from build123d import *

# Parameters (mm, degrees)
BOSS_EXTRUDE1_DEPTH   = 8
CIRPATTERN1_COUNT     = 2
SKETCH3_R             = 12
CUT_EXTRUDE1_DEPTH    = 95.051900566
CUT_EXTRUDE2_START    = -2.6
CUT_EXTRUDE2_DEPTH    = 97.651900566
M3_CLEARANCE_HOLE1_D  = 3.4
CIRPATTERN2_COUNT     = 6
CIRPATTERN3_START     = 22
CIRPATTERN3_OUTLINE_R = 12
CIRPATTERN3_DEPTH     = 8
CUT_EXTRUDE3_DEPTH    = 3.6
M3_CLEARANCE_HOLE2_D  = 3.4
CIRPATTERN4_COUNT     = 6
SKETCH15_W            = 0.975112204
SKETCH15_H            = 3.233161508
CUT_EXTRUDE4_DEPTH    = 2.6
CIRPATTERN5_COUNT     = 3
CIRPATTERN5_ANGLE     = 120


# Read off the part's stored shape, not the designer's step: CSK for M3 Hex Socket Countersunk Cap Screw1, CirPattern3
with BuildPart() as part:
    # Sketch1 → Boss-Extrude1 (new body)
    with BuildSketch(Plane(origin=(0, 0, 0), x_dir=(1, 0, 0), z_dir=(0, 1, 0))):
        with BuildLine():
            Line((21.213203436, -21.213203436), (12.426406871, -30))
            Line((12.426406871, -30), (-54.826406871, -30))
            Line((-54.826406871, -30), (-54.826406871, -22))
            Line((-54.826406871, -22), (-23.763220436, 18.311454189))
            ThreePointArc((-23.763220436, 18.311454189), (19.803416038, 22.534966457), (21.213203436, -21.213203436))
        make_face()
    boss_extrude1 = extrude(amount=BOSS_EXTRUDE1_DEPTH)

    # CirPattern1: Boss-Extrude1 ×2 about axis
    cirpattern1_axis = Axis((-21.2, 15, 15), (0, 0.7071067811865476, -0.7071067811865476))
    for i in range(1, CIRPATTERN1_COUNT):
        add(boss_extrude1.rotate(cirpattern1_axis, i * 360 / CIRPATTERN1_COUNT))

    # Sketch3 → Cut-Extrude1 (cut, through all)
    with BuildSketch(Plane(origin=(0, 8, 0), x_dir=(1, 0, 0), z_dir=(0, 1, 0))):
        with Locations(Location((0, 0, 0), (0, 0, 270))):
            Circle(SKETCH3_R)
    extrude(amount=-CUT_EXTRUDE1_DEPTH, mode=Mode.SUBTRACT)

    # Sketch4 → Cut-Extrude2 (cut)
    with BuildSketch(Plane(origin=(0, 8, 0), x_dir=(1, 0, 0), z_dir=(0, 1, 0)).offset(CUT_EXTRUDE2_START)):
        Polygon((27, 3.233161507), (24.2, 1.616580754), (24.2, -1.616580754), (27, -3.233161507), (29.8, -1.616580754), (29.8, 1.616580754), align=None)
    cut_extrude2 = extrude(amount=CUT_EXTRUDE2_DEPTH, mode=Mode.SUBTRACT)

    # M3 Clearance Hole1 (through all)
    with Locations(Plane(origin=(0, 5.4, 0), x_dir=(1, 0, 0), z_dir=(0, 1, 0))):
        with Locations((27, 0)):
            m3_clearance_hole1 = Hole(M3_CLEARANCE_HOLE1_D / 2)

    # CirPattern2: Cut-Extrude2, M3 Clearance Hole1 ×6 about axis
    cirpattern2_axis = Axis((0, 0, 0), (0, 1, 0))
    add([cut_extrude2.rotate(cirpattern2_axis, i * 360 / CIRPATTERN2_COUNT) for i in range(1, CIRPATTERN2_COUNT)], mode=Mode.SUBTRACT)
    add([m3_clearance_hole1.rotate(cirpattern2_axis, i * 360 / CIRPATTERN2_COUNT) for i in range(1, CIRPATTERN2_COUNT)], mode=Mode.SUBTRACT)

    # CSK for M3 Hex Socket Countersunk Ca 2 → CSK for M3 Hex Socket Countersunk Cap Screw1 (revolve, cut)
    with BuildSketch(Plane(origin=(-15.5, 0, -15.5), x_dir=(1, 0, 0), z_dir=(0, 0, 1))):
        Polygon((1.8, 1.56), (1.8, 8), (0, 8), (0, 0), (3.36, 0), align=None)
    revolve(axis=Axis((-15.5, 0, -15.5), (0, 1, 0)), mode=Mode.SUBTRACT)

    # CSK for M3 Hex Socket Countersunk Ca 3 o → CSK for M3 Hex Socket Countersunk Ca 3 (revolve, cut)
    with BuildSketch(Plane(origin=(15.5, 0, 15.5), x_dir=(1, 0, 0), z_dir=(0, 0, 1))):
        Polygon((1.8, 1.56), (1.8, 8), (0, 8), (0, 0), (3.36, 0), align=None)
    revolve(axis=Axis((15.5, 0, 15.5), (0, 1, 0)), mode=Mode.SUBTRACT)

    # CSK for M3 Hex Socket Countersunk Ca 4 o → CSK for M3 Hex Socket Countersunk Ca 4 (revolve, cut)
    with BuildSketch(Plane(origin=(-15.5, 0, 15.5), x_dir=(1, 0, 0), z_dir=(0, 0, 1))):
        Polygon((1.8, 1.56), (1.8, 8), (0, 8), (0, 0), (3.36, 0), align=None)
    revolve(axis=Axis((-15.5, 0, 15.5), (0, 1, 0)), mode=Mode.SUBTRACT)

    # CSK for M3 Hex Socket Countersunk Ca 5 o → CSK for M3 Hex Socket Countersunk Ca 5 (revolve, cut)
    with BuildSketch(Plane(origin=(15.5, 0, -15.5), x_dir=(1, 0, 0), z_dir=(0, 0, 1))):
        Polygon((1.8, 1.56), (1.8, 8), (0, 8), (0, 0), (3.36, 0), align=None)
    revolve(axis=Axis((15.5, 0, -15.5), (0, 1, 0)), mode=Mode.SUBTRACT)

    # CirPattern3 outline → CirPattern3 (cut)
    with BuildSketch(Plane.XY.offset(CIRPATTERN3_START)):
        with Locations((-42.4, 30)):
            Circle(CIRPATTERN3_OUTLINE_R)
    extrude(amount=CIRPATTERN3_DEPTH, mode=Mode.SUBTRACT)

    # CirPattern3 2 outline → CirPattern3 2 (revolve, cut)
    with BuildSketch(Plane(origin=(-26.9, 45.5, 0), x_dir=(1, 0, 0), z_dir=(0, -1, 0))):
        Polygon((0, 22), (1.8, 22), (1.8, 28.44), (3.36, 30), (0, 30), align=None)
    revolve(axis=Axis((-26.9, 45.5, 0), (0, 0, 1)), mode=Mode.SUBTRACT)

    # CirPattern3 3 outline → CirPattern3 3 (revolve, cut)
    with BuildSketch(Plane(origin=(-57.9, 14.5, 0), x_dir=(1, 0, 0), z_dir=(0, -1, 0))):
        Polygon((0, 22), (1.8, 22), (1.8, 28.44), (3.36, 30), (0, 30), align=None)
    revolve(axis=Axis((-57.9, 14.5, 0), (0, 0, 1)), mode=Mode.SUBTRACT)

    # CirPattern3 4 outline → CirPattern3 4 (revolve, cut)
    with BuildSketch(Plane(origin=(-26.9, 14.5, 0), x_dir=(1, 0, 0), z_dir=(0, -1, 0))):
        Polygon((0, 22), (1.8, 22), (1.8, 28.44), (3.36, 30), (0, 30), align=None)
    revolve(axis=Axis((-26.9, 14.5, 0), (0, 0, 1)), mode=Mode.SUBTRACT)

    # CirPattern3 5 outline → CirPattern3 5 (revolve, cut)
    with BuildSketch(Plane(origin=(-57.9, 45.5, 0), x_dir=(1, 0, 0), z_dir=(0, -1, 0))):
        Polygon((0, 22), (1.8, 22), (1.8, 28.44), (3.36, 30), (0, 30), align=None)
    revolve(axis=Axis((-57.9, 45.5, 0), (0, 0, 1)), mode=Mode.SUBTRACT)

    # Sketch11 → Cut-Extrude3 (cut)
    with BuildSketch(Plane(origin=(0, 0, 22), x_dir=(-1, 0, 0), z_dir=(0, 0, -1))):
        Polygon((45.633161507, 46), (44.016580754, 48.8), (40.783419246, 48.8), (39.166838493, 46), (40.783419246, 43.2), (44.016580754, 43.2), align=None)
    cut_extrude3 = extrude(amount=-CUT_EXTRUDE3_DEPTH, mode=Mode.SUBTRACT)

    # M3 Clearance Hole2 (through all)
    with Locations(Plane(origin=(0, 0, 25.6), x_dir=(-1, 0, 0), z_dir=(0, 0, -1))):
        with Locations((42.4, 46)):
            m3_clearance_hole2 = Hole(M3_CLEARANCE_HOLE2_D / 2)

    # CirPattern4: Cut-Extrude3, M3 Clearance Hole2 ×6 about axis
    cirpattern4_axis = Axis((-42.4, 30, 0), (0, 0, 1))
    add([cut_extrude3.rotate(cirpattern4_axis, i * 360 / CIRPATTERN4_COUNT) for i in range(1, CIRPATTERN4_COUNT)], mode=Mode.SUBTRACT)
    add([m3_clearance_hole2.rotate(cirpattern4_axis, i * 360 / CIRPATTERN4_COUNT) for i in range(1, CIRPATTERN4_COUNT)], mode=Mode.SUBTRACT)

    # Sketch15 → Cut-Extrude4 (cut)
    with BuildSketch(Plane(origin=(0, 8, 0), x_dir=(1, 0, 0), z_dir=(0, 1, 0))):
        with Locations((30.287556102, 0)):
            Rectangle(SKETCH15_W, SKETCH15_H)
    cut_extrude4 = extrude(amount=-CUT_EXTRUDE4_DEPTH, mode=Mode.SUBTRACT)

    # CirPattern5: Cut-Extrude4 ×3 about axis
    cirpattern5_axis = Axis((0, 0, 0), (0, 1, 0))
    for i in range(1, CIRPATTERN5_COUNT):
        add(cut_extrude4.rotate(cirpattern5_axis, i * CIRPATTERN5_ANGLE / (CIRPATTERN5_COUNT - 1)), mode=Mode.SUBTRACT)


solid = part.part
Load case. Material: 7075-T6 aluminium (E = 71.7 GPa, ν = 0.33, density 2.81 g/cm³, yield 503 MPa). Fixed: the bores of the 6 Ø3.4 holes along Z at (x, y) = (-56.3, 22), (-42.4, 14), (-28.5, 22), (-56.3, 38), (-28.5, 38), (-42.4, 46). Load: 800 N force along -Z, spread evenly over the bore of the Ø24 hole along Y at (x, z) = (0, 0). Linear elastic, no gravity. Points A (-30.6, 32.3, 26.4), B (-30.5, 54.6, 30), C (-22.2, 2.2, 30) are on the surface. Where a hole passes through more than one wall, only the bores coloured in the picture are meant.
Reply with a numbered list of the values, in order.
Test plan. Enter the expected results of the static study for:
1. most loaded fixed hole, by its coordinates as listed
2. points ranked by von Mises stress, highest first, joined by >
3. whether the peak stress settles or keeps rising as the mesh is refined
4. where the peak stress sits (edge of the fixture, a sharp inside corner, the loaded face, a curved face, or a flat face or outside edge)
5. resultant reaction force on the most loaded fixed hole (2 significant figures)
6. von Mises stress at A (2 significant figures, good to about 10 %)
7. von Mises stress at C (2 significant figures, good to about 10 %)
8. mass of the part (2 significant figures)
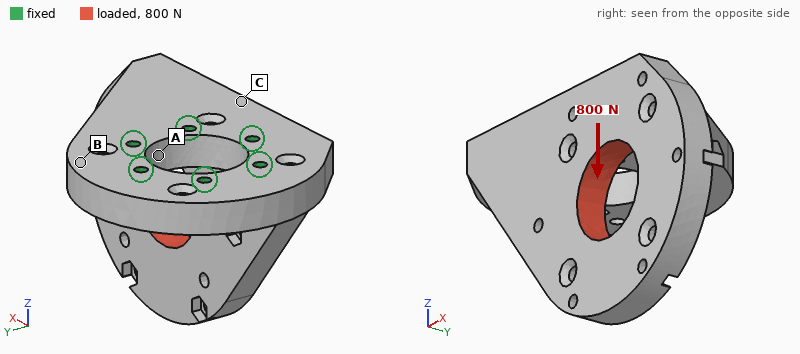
1. (-28.5, 22)
2. A > C > B
3. keeps rising
4. edge of the fixture
5. 1.5 kN
6. 25 MPa
7. 13 MPa
8. 120 g
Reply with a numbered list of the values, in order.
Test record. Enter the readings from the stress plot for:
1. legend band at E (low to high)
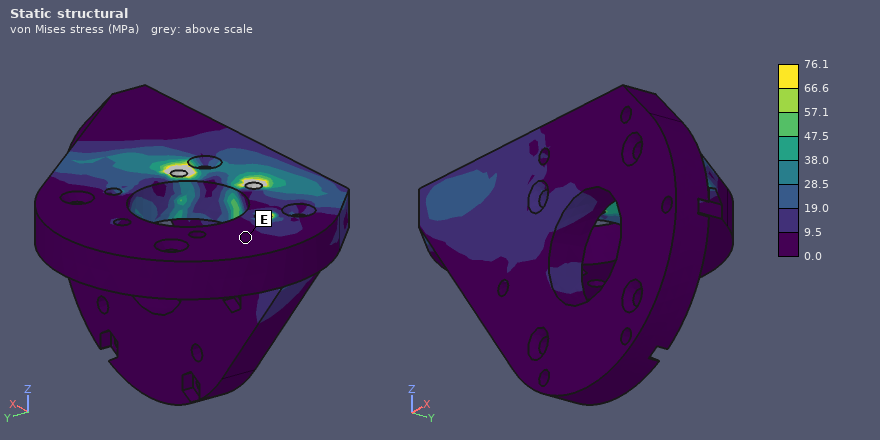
1. 0.0 to 9.5 MPa
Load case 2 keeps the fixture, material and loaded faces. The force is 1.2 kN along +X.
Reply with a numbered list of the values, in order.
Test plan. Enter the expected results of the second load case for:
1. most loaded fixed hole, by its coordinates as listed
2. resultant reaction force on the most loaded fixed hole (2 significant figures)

1. (-28.5, 22)
2. 1.4 kN
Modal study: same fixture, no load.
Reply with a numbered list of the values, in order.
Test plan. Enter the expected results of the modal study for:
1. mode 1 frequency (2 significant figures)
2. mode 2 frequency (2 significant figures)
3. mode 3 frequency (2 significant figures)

1. 1200 Hz
2. 1900 Hz
3. 4000 Hz
